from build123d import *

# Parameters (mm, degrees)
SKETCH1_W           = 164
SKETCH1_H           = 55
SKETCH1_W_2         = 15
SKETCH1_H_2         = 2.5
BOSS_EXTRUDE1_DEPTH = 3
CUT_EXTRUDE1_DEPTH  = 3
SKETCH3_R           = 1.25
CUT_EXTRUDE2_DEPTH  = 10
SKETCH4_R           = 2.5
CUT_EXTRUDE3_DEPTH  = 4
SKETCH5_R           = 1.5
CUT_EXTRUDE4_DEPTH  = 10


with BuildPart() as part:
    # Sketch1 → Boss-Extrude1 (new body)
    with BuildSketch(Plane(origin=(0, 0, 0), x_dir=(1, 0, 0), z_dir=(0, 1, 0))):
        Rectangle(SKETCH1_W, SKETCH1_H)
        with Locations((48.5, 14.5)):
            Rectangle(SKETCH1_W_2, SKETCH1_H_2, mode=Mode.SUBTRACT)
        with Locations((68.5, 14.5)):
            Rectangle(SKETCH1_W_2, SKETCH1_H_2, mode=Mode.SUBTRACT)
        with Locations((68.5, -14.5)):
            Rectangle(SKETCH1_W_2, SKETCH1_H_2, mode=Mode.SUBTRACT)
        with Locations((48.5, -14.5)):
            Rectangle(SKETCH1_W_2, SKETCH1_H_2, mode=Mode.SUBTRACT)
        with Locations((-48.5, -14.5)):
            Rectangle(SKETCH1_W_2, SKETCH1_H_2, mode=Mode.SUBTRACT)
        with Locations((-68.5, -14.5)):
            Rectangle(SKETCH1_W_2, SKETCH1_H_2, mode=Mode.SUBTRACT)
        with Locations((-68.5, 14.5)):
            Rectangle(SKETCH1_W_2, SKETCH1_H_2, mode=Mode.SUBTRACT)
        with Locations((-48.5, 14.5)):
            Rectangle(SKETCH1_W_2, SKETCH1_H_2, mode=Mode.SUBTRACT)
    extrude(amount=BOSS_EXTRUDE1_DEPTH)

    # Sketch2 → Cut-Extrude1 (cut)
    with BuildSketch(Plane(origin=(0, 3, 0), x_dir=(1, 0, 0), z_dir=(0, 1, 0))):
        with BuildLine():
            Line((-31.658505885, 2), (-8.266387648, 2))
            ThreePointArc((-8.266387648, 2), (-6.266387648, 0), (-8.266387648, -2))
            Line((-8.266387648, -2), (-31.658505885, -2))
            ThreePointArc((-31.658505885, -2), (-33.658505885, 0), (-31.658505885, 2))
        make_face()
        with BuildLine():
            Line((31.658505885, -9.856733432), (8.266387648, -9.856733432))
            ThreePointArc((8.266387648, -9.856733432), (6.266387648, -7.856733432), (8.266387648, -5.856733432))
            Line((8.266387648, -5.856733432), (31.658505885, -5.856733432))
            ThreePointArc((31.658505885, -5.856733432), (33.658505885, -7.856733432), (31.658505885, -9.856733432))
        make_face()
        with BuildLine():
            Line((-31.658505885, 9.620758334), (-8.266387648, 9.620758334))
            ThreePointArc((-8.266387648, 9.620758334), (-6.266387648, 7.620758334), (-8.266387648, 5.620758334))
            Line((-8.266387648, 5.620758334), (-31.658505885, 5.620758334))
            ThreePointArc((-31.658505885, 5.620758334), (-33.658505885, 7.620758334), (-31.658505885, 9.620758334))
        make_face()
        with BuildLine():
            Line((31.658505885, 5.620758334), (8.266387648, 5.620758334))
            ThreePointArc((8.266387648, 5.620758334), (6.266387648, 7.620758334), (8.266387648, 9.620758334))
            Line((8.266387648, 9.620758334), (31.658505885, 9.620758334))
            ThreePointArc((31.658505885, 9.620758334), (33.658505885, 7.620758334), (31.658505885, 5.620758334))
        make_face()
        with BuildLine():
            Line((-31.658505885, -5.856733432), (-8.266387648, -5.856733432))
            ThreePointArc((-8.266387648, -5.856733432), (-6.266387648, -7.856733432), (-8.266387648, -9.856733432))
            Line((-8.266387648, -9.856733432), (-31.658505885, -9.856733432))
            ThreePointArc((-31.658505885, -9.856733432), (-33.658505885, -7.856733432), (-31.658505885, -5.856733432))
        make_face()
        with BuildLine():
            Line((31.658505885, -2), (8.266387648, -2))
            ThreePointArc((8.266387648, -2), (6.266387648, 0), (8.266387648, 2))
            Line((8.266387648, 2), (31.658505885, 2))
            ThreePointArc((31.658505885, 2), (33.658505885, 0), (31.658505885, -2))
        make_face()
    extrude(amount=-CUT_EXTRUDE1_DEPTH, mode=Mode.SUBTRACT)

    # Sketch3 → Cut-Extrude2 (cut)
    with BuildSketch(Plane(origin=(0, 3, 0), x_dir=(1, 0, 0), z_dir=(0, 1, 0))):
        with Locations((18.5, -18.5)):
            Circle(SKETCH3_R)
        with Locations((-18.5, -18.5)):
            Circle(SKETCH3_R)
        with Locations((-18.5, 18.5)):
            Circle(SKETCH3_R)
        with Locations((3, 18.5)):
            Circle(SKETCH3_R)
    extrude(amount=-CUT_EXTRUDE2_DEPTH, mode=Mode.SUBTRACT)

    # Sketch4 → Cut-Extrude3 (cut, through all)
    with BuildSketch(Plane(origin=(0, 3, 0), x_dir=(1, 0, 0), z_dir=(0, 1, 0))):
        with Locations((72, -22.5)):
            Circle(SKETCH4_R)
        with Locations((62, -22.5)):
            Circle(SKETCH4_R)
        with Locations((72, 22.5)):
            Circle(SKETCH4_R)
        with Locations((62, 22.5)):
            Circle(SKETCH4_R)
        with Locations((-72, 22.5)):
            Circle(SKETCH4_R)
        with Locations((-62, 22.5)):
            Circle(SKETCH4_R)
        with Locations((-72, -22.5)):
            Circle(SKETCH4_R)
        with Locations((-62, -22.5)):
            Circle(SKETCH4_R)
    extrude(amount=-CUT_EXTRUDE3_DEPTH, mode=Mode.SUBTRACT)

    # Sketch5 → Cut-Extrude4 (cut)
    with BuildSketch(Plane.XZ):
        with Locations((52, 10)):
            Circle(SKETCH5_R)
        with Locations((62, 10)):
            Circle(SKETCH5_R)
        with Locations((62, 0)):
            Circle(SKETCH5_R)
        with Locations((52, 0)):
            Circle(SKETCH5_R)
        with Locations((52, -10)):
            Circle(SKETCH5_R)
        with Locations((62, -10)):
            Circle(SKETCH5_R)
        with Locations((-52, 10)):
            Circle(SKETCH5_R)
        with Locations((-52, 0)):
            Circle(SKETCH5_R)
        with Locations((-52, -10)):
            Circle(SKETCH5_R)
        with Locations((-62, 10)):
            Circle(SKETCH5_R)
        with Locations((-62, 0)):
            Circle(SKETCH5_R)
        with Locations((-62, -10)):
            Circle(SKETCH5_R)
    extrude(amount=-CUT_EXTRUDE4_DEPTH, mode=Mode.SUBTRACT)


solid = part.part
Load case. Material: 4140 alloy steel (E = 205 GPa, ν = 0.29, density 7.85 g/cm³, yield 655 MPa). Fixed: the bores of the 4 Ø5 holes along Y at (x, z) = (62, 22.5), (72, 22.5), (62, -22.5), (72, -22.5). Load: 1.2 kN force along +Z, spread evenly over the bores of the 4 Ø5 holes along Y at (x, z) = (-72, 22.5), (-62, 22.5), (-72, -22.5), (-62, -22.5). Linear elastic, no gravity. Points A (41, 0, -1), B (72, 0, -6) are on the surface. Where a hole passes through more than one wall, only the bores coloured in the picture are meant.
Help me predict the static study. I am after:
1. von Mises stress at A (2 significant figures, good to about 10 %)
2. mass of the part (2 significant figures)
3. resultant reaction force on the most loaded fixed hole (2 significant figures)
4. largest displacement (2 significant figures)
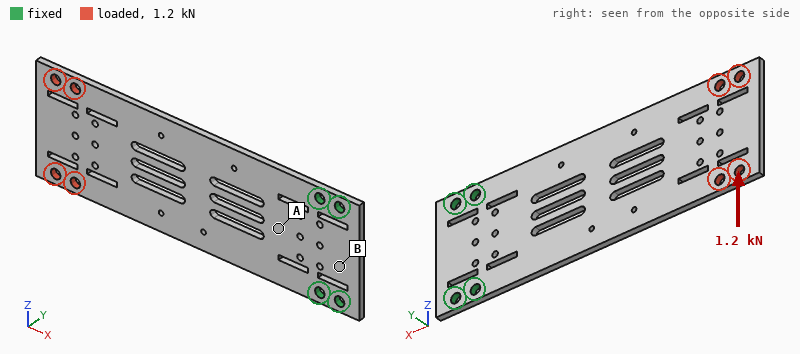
29 MPa
180 g
3.1 kN
0.18 mm
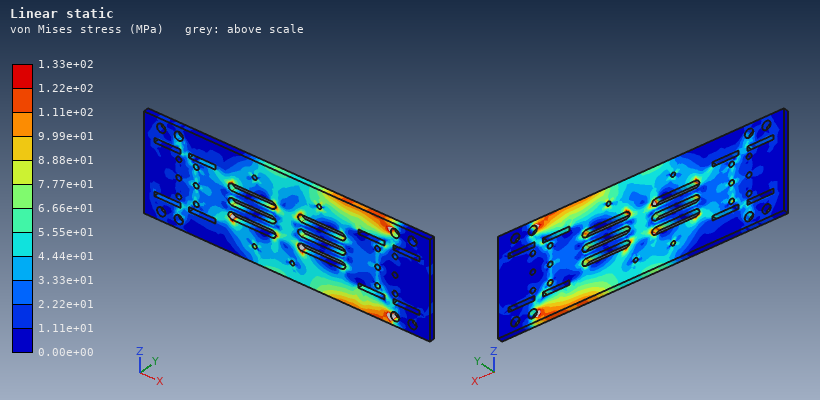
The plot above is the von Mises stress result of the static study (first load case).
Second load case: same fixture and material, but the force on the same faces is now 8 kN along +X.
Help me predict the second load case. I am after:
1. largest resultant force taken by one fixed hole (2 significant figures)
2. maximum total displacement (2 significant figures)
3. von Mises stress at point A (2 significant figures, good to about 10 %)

3.3 kN
50 µm
29 MPa
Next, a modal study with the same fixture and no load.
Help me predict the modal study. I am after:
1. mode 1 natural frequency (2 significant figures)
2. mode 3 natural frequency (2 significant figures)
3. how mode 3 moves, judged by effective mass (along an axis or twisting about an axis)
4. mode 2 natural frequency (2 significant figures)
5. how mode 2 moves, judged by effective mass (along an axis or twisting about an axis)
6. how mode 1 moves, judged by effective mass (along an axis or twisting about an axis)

120 Hz
730 Hz
along Y
610 Hz
twisting about X
along Y
